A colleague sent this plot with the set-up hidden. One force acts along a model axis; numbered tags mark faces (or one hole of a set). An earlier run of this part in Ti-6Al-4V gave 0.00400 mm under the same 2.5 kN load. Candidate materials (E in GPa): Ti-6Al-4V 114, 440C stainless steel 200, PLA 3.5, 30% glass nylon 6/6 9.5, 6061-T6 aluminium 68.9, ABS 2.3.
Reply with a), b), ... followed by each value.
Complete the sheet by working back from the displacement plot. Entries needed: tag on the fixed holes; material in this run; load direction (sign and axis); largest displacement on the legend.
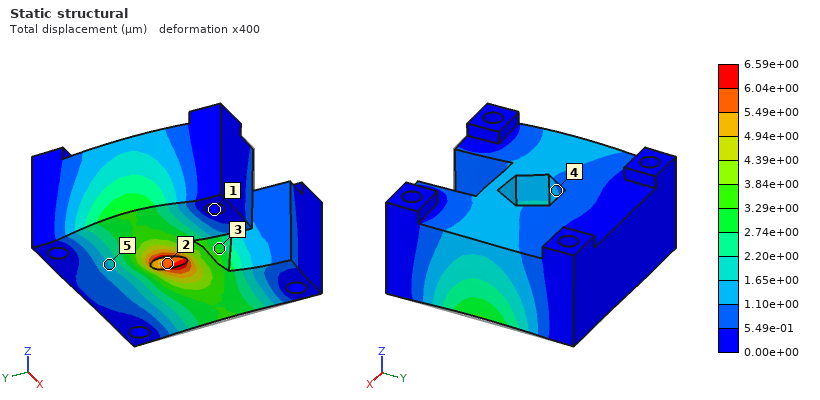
a) 1
b) 6061-T6 aluminium
c) -X
d) 6.59e+00 µm
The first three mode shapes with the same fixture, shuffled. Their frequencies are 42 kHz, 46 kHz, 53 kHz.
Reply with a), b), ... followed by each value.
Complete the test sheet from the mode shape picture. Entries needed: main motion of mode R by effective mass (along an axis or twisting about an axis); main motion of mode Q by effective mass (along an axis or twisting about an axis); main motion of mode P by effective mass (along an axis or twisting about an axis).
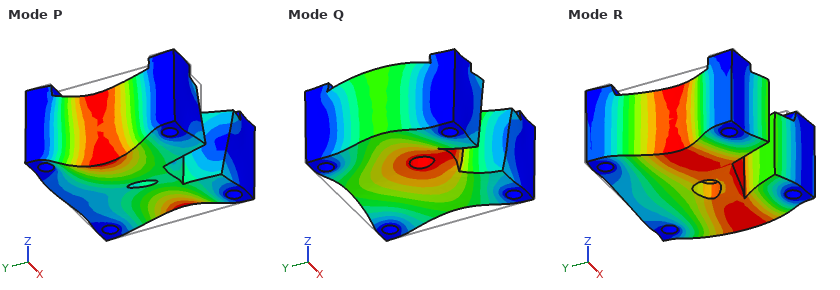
a) along X
b) along Z
c) twisting about Y
